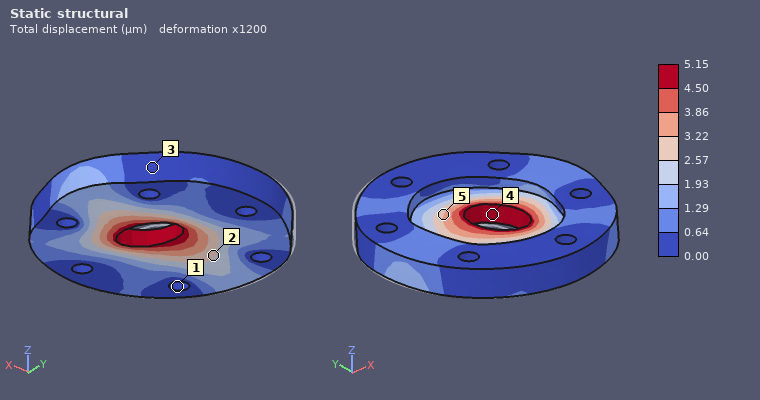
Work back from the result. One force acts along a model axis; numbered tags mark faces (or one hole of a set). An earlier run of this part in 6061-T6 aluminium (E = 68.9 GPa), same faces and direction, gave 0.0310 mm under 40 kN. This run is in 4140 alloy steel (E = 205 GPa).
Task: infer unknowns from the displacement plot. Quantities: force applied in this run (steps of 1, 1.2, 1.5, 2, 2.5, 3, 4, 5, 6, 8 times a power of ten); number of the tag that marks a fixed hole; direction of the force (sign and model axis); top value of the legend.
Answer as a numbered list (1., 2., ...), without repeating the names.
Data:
1. 20 kN
2. 1
3. +X
4. 5.15 µm
